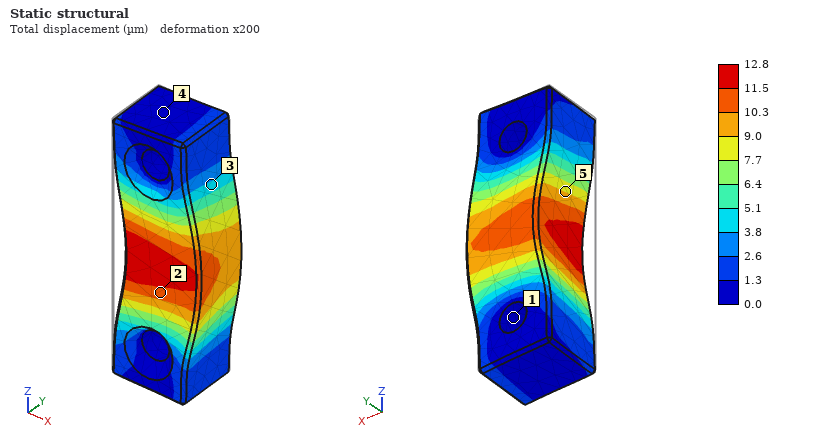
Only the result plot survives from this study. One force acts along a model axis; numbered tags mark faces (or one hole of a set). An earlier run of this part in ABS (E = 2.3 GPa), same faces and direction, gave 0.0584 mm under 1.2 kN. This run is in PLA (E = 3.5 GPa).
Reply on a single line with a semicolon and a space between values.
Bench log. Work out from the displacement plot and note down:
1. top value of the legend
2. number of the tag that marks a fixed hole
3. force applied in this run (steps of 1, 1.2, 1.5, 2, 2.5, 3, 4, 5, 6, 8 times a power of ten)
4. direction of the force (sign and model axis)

12.8 µm; 1; 400 N; +X
